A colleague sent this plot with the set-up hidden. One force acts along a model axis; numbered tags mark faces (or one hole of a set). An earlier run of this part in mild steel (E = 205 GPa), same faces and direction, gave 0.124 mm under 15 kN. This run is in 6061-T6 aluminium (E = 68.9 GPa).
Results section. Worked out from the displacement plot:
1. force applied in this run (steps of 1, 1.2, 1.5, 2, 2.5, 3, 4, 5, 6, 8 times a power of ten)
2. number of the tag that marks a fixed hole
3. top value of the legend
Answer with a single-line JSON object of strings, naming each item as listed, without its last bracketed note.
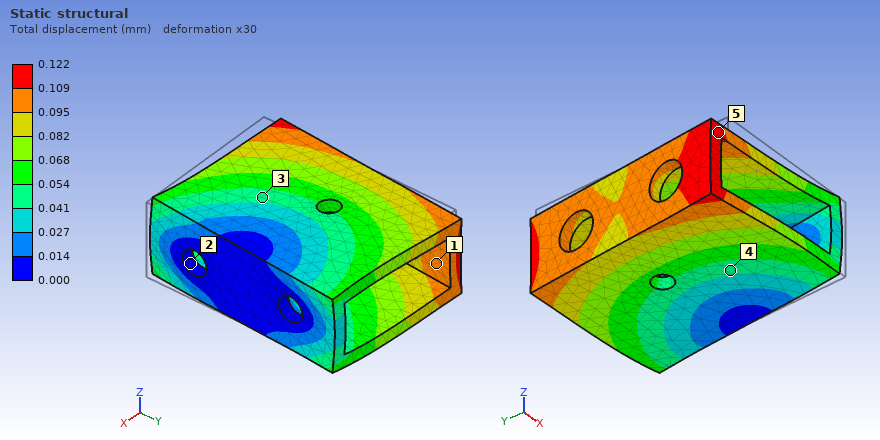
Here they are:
{"force applied in this run": "5 kN", "number of the tag that marks a fixed hole": "2", "top value of the legend": "0.122 mm"}
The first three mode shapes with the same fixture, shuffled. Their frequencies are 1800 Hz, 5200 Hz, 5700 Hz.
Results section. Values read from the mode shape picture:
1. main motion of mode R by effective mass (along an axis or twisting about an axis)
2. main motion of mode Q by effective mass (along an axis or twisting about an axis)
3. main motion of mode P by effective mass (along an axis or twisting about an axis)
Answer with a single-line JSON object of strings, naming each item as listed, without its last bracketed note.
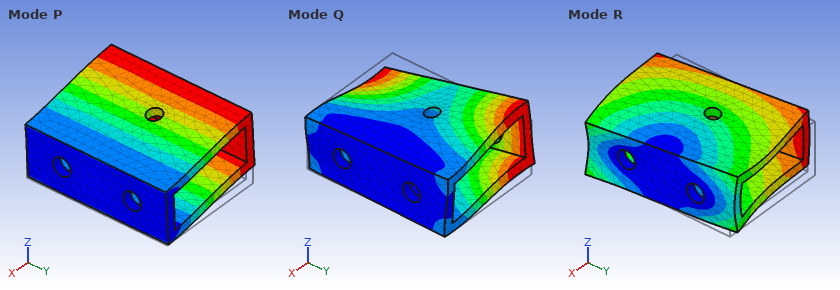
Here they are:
{"main motion of mode R by effective mass": "along Y", "main motion of mode Q by effective mass": "twisting about X", "main motion of mode P by effective mass": "along Z"}
